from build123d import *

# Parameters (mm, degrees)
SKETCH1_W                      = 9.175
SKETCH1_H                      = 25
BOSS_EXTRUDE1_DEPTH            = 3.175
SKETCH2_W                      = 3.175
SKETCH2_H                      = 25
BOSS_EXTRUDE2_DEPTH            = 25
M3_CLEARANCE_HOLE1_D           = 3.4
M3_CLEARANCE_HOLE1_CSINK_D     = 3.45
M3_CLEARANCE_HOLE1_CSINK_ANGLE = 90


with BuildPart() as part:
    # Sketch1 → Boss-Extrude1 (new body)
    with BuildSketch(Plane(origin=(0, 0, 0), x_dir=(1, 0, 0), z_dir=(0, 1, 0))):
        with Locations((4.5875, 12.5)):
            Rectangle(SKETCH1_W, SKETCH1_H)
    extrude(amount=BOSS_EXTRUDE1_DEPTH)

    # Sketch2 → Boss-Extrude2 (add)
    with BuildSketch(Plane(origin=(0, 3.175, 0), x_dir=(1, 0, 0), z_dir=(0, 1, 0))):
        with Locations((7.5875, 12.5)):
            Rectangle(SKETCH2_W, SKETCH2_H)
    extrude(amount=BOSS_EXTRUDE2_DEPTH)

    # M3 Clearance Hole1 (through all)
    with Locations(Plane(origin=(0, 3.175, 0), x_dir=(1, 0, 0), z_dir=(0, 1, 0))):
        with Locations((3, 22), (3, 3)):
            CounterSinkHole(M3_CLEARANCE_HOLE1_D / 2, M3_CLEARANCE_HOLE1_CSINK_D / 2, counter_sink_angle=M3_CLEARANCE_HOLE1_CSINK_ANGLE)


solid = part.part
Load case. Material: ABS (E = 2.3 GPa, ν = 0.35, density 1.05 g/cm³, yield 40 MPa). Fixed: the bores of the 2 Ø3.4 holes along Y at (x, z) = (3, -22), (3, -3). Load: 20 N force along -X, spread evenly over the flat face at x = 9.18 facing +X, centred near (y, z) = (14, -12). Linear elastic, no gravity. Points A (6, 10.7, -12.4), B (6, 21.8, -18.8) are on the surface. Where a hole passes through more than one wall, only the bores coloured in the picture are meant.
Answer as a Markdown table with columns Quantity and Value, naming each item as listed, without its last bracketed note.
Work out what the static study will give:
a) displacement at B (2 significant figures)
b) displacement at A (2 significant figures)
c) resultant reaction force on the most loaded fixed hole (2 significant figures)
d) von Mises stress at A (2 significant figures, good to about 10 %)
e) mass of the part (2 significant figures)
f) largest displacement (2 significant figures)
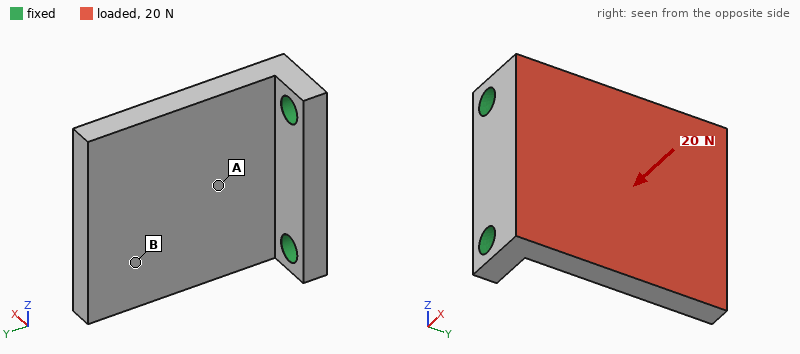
| Quantity | Value |
|---|---|
| displacement at B | 0.31 mm |
| displacement at A | 0.11 mm |
| resultant reaction force on the most loaded fixed hole | 11 N |
| von Mises stress at A | 2.5 MPa |
| mass of the part | 2.8 g |
| largest displacement | 0.44 mm |
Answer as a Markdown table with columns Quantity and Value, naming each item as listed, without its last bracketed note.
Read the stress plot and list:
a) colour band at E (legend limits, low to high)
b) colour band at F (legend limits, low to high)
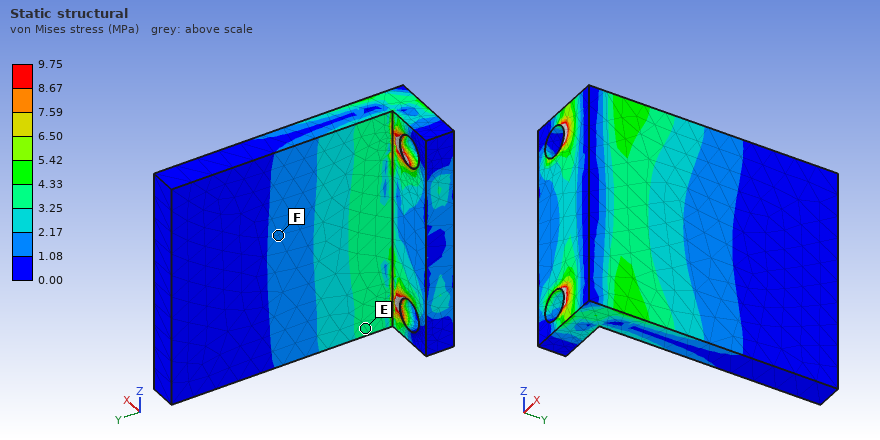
| Quantity | Value |
|---|---|
| colour band at E | 3.25 to 4.33 MPa |
| colour band at F | 1.08 to 2.17 MPa |
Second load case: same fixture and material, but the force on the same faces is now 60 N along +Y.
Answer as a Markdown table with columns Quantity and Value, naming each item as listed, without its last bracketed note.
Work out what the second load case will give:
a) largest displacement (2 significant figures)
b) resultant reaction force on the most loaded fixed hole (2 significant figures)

| Quantity | Value |
|---|---|
| largest displacement | 0.31 mm |
| resultant reaction force on the most loaded fixed hole | 30 N |
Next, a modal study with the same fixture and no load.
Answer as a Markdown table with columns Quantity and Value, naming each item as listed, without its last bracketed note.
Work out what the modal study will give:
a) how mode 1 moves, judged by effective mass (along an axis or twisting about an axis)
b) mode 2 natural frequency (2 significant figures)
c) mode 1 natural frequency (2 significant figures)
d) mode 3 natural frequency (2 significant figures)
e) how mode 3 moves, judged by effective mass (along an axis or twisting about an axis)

| Quantity | Value |
|---|---|
| how mode 1 moves, judged by effective mass | along X |
| mode 2 natural frequency | 2400 Hz |
| mode 1 natural frequency | 870 Hz |
| mode 3 natural frequency | 3700 Hz |
| how mode 3 moves, judged by effective mass | along Z |
